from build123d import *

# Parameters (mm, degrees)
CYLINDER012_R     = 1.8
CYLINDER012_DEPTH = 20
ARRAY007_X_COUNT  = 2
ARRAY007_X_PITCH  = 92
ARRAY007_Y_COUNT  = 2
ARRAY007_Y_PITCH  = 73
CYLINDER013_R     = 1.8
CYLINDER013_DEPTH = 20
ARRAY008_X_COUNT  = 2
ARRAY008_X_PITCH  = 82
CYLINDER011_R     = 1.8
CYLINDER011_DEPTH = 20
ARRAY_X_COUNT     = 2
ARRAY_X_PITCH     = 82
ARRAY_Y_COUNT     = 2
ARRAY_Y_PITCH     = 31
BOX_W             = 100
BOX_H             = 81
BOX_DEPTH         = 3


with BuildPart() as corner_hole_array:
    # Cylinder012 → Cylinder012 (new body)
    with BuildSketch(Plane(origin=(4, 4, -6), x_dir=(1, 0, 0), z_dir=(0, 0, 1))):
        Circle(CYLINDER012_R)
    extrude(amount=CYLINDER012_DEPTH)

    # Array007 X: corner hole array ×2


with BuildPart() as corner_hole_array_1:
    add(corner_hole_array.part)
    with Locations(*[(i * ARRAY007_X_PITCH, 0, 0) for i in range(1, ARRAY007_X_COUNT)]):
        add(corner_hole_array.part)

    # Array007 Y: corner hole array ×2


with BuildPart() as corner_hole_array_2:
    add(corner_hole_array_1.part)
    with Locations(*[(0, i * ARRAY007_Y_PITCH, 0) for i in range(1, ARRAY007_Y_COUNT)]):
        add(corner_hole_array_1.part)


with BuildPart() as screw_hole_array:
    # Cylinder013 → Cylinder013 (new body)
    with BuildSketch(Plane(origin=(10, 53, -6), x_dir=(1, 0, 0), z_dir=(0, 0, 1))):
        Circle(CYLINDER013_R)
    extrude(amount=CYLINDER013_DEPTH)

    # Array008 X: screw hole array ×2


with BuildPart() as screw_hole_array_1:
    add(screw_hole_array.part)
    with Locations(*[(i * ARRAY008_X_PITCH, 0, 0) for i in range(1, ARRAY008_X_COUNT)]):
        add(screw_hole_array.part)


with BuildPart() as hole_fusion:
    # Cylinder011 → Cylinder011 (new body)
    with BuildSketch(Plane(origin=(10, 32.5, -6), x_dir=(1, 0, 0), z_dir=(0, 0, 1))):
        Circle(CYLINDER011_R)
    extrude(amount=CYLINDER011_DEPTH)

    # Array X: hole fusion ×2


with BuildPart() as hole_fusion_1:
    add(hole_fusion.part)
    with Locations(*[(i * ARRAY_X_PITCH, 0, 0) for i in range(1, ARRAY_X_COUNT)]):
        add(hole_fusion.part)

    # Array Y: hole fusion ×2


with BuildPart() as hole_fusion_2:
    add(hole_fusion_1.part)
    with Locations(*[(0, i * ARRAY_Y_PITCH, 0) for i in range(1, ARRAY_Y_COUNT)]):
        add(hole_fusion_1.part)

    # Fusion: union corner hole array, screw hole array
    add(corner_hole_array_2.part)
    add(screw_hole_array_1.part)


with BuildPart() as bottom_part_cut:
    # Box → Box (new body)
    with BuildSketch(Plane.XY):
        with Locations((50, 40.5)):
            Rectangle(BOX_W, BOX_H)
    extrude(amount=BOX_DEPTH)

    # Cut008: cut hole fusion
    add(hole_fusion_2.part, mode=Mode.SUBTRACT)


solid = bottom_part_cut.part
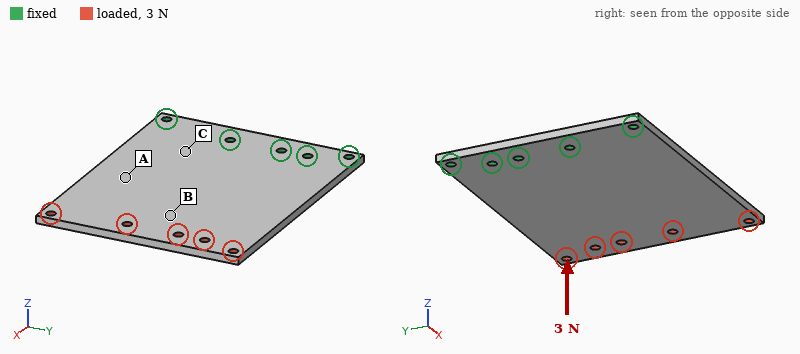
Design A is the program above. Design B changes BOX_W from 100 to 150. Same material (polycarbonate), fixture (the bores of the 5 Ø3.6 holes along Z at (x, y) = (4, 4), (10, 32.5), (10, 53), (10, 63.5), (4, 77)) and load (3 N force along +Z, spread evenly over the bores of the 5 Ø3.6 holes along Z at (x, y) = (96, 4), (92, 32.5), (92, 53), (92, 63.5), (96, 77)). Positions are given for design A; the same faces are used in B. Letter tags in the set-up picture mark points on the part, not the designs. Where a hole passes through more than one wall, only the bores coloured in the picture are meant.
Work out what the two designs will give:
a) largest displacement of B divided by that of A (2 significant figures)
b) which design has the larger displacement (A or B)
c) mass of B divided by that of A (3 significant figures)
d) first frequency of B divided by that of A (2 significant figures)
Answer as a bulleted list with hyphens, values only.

- 1.4
- B
- 1.51
- 0.61
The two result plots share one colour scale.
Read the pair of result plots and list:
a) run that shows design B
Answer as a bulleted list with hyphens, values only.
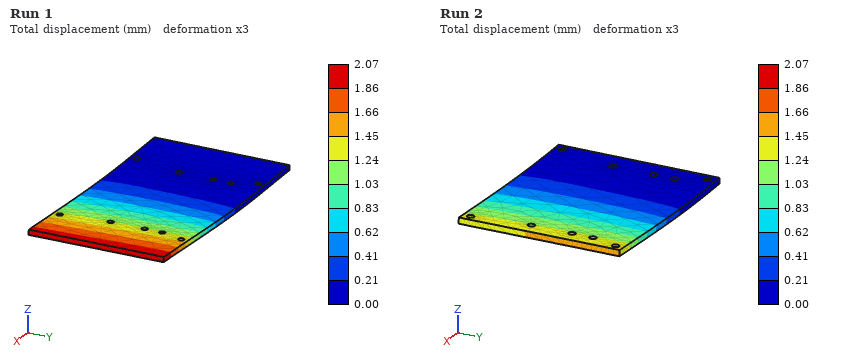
- Run 1
